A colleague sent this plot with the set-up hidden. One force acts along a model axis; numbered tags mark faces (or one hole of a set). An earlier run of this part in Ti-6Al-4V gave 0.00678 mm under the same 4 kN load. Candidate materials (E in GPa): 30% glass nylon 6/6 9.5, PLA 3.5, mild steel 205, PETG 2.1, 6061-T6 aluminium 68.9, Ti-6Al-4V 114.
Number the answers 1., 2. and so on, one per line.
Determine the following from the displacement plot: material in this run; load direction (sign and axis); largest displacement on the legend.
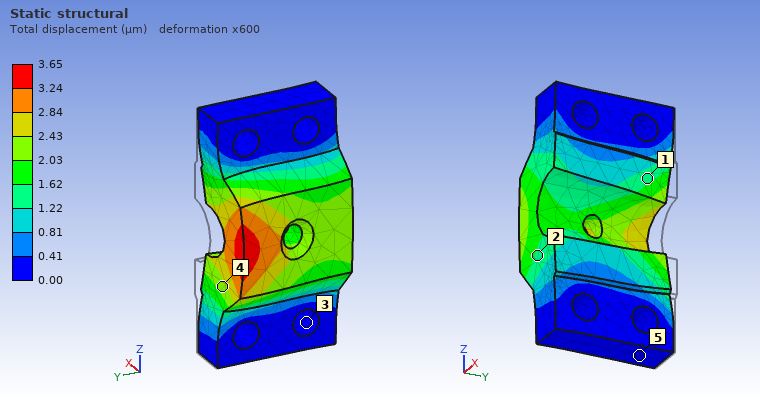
1. mild steel
2. -Y
3. 3.65 µm
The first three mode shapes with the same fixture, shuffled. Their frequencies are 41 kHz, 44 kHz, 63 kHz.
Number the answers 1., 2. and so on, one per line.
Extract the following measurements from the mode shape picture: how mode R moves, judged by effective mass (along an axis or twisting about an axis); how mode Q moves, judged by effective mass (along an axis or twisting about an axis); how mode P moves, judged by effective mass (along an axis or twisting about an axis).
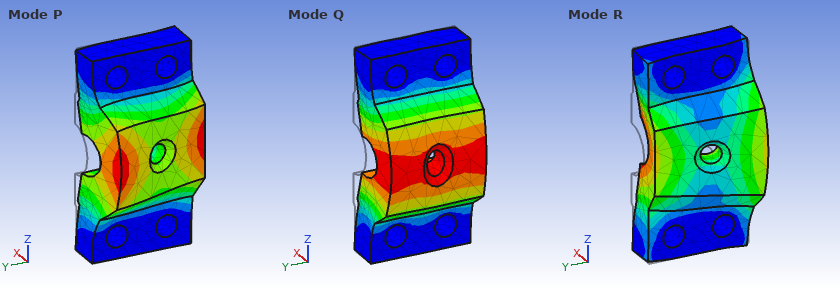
1. along Y
2. along X
3. along Y
